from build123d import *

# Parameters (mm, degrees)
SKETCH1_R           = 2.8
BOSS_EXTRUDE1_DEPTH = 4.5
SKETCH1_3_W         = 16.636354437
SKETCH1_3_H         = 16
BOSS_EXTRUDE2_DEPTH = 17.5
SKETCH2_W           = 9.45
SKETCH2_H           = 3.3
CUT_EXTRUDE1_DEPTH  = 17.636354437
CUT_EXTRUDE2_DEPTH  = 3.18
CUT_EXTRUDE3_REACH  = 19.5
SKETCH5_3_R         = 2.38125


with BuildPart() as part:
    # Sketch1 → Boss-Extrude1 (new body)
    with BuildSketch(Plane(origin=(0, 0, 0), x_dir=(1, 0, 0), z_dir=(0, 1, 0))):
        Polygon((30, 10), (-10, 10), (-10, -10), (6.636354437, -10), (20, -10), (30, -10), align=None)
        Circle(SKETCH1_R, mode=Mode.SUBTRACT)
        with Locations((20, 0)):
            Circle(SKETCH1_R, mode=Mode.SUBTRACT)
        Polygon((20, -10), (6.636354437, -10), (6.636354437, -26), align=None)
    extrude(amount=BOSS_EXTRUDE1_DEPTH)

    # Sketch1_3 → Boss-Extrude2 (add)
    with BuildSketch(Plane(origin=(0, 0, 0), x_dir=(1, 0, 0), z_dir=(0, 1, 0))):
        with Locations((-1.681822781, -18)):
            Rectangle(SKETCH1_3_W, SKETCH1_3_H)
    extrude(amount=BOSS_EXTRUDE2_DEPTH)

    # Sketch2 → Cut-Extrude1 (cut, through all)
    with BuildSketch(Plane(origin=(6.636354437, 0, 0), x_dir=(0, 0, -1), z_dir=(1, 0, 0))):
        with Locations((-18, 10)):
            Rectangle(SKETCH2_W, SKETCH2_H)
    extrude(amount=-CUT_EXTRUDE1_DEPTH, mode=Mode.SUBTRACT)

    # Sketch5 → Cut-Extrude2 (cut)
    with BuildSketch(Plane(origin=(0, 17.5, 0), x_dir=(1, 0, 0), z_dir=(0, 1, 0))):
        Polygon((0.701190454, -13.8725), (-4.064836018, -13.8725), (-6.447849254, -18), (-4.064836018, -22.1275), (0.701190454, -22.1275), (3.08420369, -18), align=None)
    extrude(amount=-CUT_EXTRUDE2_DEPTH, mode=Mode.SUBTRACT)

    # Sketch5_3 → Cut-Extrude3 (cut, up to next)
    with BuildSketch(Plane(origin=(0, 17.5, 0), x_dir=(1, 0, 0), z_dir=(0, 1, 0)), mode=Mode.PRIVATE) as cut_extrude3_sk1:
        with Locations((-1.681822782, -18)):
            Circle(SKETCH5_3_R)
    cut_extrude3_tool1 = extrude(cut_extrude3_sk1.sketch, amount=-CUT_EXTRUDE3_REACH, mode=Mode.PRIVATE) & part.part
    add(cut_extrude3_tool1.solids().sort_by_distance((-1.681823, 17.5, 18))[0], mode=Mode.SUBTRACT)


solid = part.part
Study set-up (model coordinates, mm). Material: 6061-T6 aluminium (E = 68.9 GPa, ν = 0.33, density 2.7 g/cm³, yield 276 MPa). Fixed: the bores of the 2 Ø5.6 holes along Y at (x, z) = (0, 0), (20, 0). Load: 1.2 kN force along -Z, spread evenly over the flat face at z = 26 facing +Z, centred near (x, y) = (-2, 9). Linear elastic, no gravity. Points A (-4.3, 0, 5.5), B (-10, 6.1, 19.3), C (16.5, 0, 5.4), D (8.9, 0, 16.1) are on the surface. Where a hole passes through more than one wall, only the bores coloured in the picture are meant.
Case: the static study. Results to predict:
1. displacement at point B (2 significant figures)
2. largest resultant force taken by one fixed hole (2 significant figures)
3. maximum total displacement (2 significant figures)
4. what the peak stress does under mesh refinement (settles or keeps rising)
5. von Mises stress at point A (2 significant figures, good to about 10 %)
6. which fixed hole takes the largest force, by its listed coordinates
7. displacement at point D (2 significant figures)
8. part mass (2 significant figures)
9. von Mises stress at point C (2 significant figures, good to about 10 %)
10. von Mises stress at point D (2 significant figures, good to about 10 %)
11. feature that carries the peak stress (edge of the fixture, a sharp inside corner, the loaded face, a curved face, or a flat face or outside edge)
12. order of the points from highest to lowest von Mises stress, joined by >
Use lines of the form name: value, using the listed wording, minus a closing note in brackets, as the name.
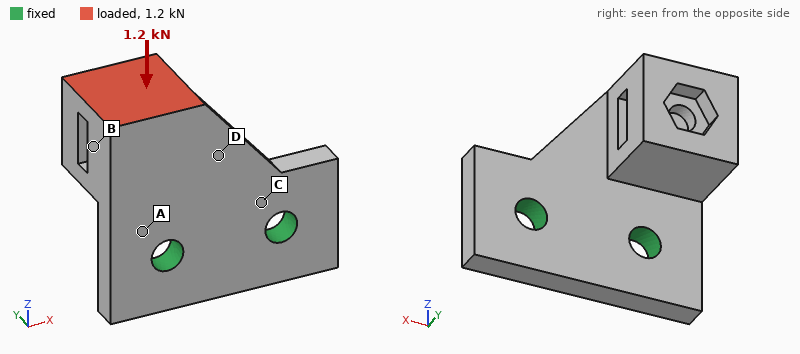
displacement at point B: 0.086 mm
largest resultant force taken by one fixed hole: 1.2 kN
maximum total displacement: 0.16 mm
what the peak stress does under mesh refinement: keeps rising
von Mises stress at point A: 63 MPa
which fixed hole takes the largest force, by its listed coordinates: (0, 0)
displacement at point D: 0.050 mm
part mass: 21 g
von Mises stress at point C: 52 MPa
von Mises stress at point D: 35 MPa
feature that carries the peak stress: edge of the fixture
order of the points from highest to lowest von Mises stress, joined by >: A > C > D > B
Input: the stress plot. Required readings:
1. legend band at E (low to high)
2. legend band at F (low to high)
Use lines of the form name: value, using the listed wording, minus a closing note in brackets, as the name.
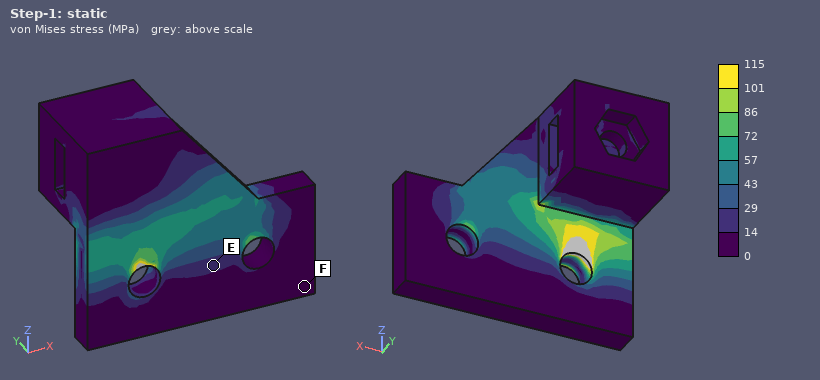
legend band at E: 14 to 29 MPa
legend band at F: 0 to 14 MPa
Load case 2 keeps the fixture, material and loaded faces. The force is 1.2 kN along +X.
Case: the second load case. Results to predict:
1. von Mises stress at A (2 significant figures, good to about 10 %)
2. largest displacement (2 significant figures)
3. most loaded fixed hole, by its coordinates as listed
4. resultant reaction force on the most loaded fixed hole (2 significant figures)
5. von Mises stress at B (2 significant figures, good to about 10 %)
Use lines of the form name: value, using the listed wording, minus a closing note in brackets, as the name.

von Mises stress at A: 53 MPa
largest displacement: 77 µm
most loaded fixed hole, by its coordinates as listed: (20, 0)
resultant reaction force on the most loaded fixed hole: 1.5 kN
von Mises stress at B: 23 MPa
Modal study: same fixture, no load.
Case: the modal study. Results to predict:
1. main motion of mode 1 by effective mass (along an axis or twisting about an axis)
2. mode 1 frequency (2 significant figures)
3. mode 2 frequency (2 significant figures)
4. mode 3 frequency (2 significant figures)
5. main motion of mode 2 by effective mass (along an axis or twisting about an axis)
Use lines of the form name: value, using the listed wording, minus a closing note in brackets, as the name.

main motion of mode 1 by effective mass: along Y
mode 1 frequency: 3600 Hz
mode 2 frequency: 8300 Hz
mode 3 frequency: 17 kHz
main motion of mode 2 by effective mass: along X
